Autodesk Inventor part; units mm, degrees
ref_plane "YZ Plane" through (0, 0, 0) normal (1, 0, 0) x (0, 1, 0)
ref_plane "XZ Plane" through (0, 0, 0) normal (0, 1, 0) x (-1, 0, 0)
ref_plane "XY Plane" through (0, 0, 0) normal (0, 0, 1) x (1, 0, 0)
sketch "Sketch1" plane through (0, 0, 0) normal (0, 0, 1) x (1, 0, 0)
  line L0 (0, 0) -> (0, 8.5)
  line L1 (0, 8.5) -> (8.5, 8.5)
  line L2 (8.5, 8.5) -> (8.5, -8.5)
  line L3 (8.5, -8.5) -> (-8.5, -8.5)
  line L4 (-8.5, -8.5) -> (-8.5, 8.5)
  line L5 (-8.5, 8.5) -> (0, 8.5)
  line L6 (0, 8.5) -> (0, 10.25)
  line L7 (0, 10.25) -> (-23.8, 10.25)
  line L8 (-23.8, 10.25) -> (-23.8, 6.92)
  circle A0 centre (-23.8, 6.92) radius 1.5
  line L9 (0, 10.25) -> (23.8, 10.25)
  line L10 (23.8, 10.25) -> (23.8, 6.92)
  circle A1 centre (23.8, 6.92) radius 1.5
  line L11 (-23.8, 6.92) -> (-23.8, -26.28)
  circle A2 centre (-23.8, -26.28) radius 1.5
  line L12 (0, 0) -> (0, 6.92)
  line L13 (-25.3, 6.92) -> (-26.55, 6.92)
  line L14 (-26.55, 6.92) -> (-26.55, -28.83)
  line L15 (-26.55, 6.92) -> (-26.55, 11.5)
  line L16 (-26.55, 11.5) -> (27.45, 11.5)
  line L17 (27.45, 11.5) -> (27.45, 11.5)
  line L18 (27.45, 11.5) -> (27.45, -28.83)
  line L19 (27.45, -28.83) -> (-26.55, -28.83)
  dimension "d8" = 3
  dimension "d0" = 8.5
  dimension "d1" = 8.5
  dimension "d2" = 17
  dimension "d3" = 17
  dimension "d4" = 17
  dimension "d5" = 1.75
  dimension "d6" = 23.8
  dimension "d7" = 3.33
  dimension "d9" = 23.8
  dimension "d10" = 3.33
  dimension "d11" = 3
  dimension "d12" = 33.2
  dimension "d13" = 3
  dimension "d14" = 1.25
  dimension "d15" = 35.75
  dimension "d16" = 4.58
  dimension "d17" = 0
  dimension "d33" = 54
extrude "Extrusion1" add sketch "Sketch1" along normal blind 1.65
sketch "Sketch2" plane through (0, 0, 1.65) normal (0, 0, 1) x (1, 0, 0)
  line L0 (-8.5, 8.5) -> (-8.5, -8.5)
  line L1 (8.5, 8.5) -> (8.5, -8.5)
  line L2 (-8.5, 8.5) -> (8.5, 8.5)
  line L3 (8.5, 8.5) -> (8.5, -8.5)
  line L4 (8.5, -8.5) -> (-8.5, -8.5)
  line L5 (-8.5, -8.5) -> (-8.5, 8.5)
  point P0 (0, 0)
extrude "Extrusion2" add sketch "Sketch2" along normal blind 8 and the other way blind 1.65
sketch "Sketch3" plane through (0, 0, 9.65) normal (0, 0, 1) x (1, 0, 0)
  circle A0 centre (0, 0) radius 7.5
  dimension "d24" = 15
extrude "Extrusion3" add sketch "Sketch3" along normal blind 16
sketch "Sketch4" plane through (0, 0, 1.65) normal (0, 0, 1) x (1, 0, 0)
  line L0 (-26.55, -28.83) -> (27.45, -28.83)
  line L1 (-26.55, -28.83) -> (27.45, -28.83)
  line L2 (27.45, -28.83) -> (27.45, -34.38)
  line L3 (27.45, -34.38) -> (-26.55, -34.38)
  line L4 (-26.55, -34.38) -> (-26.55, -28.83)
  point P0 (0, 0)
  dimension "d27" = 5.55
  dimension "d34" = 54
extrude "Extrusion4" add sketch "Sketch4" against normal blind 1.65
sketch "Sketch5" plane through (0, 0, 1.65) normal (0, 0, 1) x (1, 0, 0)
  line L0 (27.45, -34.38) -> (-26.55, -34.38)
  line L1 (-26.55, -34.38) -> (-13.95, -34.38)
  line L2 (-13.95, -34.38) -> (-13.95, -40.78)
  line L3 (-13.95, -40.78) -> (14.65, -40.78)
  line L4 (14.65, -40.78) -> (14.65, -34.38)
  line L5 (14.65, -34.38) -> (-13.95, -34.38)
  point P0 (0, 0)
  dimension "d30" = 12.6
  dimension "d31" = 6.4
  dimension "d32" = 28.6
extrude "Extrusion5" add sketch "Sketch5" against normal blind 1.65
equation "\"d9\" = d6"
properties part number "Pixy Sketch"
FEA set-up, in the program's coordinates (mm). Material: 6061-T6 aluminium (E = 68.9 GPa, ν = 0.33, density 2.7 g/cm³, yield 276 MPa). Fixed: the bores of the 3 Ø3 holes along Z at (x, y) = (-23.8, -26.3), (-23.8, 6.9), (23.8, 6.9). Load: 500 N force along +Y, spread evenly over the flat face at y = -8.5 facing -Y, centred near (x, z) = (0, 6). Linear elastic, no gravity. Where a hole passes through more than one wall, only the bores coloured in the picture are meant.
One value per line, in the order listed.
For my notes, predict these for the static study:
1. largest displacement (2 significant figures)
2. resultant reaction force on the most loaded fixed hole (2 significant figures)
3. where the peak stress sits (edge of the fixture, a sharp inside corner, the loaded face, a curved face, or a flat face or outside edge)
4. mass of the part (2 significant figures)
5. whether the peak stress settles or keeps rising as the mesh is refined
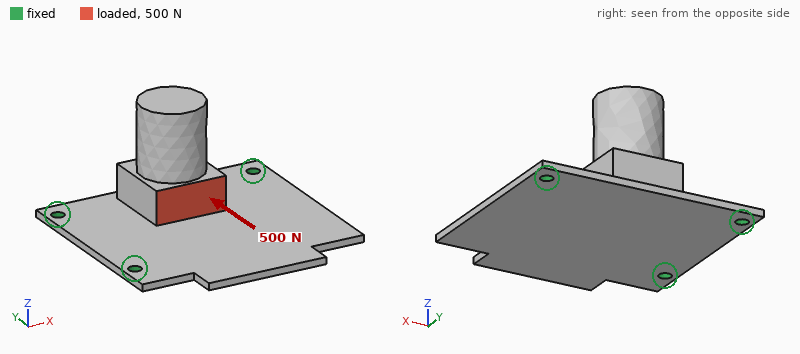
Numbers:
0.23 mm
220 N
edge of the fixture
26 g
keeps rising
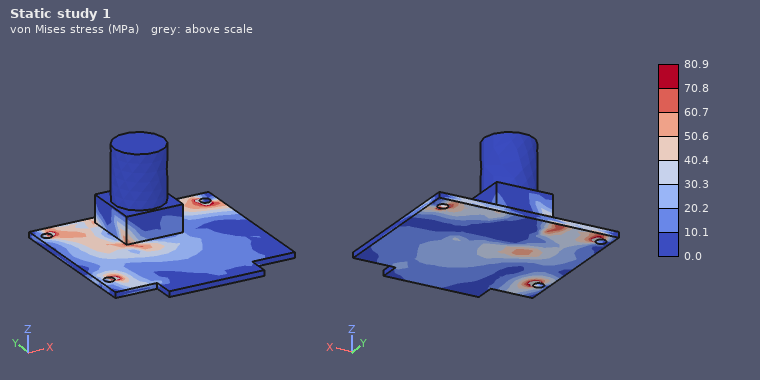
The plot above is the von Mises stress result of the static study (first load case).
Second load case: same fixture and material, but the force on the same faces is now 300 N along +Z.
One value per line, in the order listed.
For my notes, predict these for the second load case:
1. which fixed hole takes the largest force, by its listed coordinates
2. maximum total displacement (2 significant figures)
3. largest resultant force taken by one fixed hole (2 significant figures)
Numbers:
(23.8, 6.9)
0.38 mm
140 N
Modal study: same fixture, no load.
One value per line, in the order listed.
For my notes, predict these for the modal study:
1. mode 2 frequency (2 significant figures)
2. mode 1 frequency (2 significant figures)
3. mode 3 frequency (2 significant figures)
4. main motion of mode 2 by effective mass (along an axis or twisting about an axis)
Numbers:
2100 Hz
1100 Hz
2300 Hz
along Z
